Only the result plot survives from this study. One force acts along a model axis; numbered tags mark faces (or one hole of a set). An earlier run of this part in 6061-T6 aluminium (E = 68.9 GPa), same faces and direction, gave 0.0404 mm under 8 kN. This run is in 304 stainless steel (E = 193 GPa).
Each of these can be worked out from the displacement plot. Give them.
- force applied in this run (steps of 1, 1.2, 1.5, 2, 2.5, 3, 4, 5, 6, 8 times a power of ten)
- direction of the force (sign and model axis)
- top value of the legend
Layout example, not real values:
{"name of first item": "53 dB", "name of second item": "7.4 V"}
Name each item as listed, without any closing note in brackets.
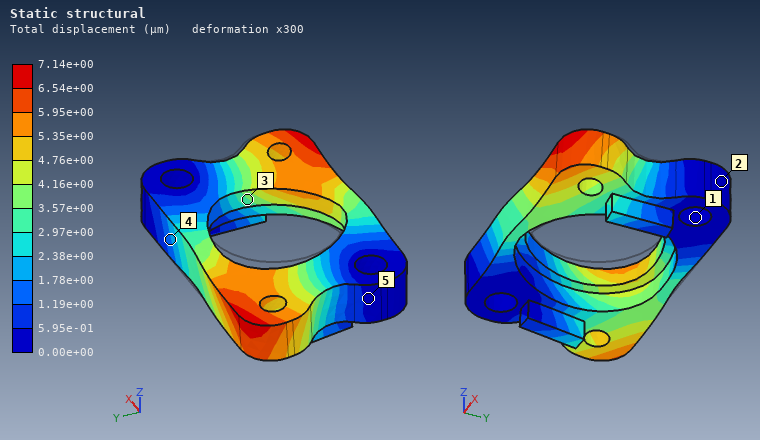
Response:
{"force applied in this run": "4 kN", "direction of the force": "-X", "top value of the legend": "7.14e+00 µm"}
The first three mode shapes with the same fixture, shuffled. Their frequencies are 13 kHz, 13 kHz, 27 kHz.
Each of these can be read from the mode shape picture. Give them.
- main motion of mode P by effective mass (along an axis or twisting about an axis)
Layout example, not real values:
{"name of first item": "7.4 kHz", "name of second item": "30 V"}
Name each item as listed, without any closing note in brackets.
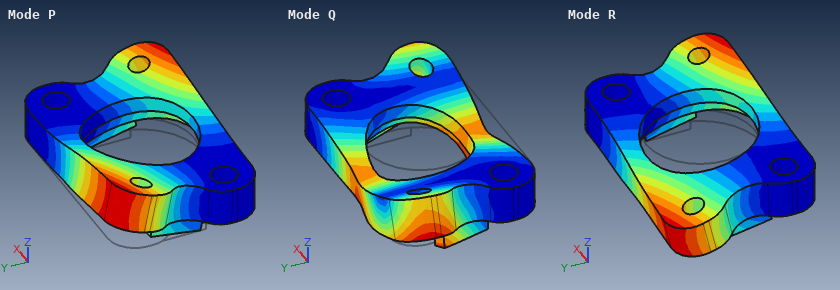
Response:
{"main motion of mode P by effective mass": "along Z"}
